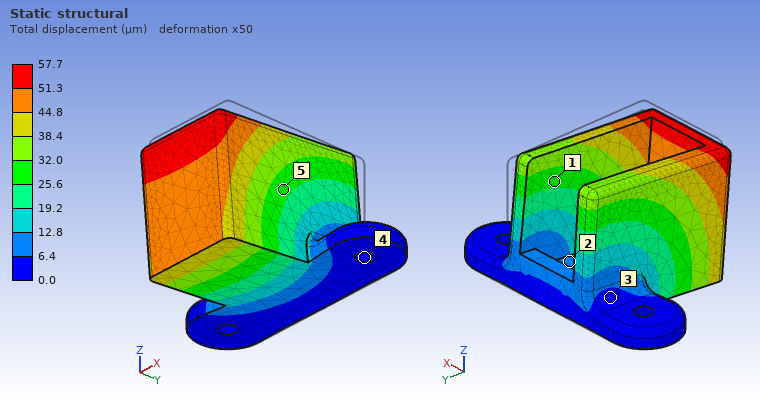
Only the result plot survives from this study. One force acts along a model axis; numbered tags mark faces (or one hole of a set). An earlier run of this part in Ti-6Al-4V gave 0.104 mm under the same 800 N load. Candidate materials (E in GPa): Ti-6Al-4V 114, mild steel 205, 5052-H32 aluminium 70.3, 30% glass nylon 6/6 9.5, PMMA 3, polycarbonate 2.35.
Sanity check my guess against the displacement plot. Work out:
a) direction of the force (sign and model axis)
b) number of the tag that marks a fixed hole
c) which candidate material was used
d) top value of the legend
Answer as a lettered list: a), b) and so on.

a) -Z
b) 4
c) mild steel
d) 57.7 µm
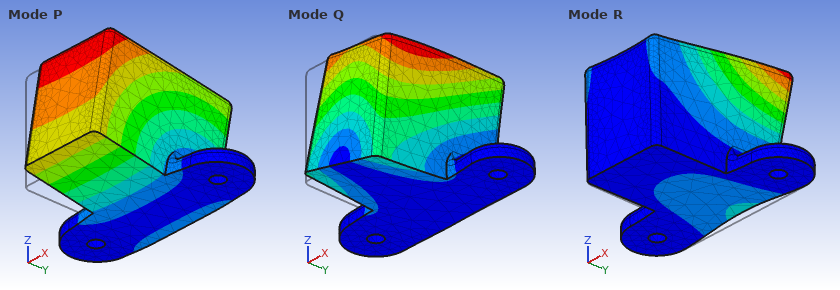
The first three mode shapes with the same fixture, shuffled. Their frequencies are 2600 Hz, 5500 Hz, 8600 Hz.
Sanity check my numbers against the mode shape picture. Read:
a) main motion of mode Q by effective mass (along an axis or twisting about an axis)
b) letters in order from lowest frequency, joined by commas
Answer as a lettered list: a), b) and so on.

a) along X
b) P, Q, R
